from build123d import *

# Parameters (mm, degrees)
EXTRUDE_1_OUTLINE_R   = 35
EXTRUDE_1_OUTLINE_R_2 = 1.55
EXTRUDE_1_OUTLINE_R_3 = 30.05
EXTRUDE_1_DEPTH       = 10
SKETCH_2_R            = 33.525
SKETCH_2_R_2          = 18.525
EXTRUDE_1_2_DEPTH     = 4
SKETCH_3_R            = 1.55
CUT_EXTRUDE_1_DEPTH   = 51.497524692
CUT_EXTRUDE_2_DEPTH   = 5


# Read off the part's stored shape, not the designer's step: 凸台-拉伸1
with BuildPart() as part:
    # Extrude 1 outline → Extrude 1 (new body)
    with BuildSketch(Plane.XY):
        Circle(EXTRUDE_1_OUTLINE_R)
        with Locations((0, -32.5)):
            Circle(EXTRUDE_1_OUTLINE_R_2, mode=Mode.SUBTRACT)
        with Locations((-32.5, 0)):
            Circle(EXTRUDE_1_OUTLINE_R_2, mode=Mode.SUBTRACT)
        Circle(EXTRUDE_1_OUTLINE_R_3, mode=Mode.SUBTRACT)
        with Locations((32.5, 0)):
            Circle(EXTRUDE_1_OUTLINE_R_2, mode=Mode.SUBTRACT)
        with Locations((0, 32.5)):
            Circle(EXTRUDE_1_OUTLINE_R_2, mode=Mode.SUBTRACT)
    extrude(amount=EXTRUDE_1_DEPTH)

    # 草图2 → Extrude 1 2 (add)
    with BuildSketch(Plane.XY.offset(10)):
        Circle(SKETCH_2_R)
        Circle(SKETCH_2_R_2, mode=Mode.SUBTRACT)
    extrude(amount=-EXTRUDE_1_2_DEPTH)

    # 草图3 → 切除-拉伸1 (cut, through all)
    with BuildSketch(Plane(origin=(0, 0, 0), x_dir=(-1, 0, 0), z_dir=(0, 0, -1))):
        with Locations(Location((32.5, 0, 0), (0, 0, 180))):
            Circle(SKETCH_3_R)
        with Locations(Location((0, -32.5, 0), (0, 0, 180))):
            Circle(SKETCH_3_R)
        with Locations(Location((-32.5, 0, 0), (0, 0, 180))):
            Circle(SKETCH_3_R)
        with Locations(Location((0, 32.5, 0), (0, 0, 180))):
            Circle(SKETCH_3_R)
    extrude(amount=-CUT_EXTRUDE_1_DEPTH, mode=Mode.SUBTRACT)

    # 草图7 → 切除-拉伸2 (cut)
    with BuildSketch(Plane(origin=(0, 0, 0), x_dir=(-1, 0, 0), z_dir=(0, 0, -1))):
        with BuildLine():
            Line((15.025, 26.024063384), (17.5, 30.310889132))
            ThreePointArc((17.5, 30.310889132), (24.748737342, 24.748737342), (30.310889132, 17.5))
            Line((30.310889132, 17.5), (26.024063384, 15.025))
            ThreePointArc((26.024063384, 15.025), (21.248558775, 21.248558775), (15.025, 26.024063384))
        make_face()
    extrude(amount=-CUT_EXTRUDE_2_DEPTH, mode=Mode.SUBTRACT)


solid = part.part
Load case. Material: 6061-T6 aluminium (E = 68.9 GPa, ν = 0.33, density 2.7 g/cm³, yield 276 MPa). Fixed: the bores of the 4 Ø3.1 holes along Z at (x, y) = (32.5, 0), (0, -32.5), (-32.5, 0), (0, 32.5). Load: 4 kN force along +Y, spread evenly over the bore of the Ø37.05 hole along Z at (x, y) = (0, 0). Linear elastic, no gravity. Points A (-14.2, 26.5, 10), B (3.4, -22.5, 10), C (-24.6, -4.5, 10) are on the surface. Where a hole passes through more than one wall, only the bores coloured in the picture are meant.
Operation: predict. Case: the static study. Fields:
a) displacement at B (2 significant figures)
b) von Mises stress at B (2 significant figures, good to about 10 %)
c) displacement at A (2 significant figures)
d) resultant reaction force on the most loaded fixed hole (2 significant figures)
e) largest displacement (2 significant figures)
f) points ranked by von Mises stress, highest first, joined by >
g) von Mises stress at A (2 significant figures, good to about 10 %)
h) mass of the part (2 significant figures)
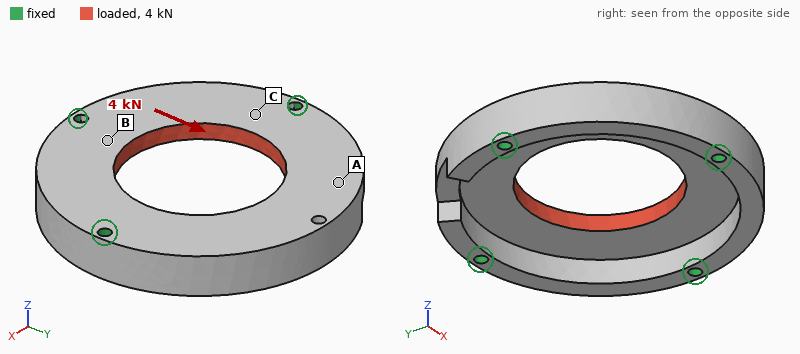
7.2 µm
19 MPa
7.0 µm
1.2 kN
9.9 µm
B > A > C
10 MPa
44 g
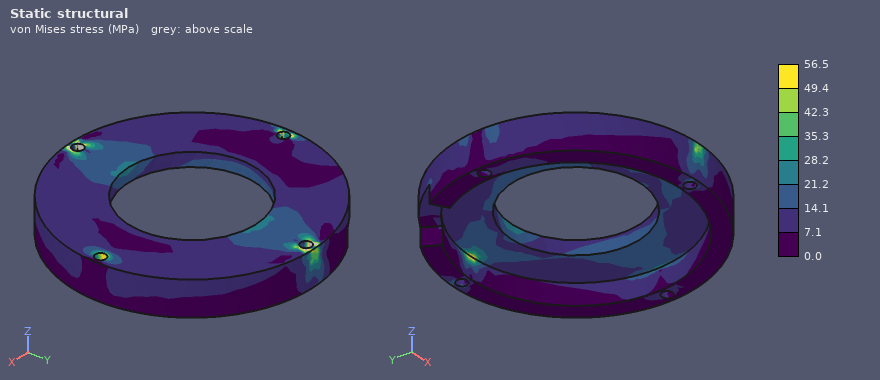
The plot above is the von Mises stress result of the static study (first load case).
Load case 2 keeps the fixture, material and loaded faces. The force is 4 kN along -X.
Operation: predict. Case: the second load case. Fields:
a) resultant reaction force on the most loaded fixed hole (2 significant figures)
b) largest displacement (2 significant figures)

1.1 kN
9.2 µm
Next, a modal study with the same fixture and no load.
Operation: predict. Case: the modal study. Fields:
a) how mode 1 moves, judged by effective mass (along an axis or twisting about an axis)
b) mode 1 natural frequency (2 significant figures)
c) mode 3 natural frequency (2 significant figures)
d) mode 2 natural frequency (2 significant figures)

along Z
12 kHz
14 kHz
13 kHz
